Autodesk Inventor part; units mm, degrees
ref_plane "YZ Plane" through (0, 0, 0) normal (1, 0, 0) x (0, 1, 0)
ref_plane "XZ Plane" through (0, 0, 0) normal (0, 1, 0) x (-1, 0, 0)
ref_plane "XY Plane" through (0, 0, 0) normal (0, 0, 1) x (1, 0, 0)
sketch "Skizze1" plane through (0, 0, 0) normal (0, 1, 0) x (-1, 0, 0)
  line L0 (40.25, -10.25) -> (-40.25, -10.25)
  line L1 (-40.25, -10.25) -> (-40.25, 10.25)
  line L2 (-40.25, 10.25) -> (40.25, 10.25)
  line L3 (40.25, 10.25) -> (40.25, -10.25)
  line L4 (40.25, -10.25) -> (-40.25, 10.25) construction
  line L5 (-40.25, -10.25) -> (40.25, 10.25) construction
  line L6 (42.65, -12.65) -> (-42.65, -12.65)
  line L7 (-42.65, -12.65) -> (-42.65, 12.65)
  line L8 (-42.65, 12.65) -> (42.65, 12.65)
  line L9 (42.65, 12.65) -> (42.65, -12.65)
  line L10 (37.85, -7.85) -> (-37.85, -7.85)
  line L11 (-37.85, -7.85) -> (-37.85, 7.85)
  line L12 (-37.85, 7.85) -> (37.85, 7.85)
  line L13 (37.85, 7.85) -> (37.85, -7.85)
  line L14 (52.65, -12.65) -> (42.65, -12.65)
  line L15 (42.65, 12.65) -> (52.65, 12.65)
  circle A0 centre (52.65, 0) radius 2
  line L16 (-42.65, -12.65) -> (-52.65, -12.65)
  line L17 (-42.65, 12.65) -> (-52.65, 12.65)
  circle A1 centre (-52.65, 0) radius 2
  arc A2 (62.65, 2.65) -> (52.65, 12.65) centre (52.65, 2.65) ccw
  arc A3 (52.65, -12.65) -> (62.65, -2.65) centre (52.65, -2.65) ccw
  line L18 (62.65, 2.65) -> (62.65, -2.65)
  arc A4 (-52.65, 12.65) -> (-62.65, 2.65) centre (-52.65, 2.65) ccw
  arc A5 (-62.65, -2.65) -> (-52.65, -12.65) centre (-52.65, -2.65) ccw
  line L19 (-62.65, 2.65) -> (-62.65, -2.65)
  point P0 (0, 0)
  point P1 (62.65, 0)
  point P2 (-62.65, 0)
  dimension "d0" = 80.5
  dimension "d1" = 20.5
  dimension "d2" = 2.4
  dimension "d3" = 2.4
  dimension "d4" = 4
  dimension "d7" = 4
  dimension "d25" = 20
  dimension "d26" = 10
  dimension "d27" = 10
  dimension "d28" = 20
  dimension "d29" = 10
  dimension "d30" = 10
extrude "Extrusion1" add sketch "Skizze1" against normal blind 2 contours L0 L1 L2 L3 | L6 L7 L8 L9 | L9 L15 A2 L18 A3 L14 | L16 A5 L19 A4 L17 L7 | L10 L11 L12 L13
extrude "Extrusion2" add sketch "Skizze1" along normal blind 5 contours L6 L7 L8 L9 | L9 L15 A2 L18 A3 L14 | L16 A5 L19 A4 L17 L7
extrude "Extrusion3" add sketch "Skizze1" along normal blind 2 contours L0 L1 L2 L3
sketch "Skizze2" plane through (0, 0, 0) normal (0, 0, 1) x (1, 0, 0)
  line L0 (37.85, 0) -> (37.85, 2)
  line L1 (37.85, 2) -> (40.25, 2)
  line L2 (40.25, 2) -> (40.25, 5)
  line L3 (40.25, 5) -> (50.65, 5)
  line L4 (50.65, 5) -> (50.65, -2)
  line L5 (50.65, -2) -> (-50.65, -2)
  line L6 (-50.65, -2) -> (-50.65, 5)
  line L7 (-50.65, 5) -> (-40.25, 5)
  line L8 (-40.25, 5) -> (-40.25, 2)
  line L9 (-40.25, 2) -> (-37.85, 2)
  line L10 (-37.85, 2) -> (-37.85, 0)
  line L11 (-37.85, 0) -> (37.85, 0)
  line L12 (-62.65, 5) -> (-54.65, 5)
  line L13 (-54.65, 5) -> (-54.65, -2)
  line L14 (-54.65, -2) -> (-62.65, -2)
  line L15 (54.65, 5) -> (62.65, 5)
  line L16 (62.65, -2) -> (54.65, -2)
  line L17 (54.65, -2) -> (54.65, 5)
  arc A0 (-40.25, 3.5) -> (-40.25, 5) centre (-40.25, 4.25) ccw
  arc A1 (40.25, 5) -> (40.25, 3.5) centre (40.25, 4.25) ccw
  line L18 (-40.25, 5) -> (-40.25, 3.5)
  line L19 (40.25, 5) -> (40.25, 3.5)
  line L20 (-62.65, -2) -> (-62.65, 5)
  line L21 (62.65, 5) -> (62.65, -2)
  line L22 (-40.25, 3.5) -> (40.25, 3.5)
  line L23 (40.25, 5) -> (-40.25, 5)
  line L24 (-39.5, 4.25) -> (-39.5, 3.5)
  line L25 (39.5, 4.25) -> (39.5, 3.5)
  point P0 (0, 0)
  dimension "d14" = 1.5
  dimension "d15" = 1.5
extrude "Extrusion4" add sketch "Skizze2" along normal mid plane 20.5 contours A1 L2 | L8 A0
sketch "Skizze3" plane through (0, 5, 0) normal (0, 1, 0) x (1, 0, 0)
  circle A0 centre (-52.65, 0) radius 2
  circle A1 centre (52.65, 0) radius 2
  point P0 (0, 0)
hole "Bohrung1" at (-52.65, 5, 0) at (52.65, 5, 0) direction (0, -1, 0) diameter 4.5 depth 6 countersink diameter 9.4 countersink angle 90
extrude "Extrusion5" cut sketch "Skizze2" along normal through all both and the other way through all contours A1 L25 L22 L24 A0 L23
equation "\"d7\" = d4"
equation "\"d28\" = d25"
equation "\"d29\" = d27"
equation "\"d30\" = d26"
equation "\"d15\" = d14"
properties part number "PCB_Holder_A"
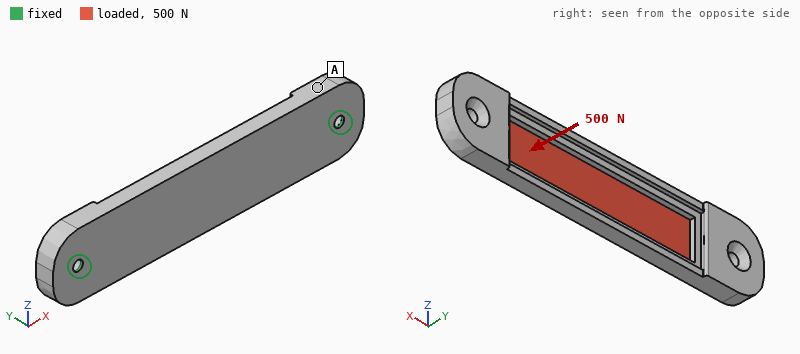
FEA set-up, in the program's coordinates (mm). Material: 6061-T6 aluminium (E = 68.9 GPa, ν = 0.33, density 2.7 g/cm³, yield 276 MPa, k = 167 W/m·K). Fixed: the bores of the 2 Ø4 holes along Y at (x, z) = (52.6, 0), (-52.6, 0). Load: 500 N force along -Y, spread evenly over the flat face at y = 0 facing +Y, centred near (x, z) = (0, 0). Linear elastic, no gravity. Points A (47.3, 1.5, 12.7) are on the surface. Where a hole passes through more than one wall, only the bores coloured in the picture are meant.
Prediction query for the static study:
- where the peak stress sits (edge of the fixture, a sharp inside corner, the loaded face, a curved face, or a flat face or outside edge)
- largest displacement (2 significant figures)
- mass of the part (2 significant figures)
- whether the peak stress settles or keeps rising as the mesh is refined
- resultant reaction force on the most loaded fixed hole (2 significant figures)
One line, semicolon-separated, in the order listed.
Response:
edge of the fixture; 0.28 mm; 36 g; keeps rising; 640 N
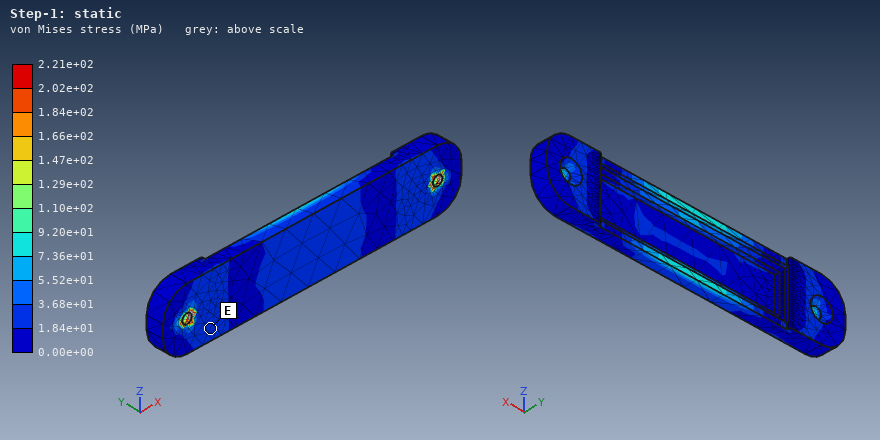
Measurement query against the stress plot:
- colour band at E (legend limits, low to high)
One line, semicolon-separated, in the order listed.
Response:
1.84e+01 to 3.68e+01 MPa
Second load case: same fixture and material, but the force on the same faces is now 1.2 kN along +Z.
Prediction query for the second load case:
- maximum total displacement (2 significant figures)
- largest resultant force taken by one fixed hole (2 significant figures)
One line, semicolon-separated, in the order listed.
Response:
92 µm; 600 N
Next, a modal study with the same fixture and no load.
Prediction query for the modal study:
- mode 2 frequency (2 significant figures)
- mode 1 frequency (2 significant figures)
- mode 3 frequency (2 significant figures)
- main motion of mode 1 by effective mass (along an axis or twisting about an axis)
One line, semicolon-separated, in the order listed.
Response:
3200 Hz; 1800 Hz; 4500 Hz; along Y
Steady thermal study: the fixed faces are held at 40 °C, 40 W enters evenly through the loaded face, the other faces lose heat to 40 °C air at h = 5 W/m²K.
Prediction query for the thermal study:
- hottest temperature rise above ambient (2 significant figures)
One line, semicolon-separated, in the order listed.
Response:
53 K
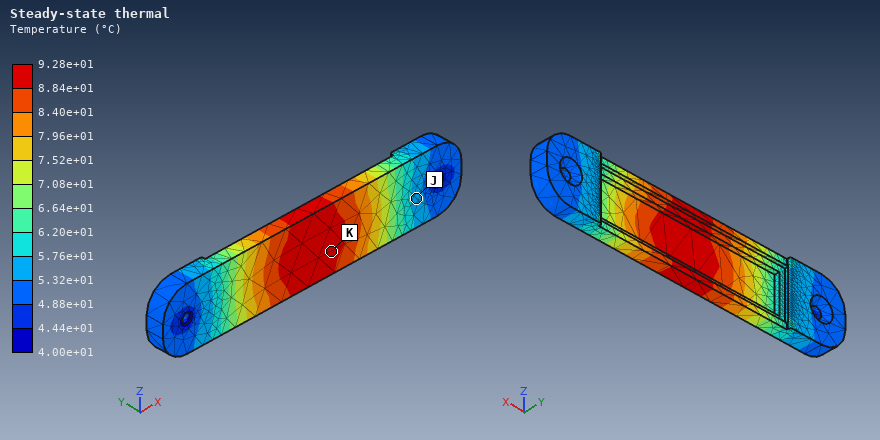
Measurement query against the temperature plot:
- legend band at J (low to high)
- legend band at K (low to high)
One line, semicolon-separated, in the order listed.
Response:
5.32e+01 to 5.76e+01 °C; 8.84e+01 to 9.28e+01 °C
